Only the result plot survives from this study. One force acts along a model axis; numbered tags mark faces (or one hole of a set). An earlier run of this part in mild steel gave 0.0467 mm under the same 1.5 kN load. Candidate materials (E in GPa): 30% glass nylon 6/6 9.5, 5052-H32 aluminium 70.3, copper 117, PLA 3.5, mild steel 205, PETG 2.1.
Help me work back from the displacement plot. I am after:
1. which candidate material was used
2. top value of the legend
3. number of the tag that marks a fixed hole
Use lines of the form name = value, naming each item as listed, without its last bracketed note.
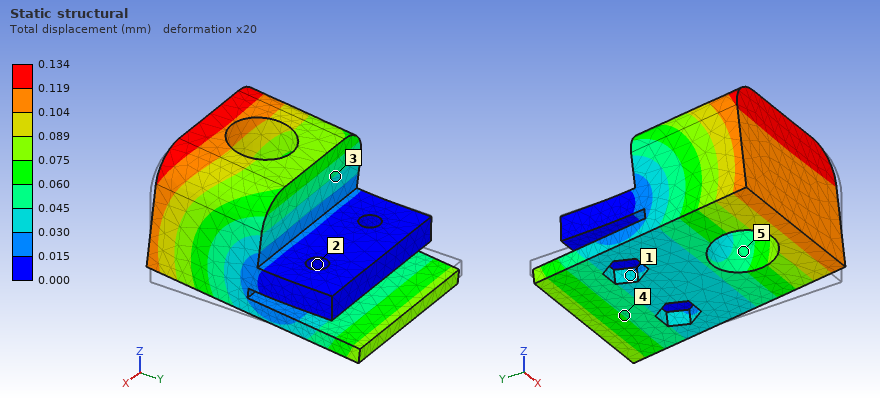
which candidate material was used = 5052-H32 aluminium
top value of the legend = 0.134 mm
number of the tag that marks a fixed hole = 2
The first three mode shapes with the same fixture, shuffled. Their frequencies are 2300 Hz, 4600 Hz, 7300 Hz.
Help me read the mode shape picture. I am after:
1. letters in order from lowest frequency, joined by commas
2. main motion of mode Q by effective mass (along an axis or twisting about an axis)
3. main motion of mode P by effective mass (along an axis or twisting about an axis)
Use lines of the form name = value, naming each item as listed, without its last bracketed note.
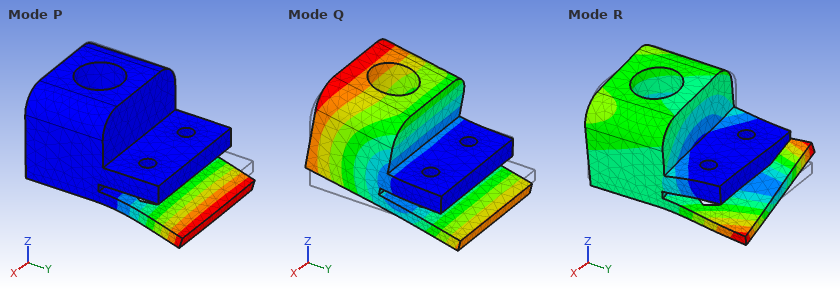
letters in order from lowest frequency, joined by commas = Q, P, R
main motion of mode Q by effective mass = along Z
main motion of mode P by effective mass = along Z
